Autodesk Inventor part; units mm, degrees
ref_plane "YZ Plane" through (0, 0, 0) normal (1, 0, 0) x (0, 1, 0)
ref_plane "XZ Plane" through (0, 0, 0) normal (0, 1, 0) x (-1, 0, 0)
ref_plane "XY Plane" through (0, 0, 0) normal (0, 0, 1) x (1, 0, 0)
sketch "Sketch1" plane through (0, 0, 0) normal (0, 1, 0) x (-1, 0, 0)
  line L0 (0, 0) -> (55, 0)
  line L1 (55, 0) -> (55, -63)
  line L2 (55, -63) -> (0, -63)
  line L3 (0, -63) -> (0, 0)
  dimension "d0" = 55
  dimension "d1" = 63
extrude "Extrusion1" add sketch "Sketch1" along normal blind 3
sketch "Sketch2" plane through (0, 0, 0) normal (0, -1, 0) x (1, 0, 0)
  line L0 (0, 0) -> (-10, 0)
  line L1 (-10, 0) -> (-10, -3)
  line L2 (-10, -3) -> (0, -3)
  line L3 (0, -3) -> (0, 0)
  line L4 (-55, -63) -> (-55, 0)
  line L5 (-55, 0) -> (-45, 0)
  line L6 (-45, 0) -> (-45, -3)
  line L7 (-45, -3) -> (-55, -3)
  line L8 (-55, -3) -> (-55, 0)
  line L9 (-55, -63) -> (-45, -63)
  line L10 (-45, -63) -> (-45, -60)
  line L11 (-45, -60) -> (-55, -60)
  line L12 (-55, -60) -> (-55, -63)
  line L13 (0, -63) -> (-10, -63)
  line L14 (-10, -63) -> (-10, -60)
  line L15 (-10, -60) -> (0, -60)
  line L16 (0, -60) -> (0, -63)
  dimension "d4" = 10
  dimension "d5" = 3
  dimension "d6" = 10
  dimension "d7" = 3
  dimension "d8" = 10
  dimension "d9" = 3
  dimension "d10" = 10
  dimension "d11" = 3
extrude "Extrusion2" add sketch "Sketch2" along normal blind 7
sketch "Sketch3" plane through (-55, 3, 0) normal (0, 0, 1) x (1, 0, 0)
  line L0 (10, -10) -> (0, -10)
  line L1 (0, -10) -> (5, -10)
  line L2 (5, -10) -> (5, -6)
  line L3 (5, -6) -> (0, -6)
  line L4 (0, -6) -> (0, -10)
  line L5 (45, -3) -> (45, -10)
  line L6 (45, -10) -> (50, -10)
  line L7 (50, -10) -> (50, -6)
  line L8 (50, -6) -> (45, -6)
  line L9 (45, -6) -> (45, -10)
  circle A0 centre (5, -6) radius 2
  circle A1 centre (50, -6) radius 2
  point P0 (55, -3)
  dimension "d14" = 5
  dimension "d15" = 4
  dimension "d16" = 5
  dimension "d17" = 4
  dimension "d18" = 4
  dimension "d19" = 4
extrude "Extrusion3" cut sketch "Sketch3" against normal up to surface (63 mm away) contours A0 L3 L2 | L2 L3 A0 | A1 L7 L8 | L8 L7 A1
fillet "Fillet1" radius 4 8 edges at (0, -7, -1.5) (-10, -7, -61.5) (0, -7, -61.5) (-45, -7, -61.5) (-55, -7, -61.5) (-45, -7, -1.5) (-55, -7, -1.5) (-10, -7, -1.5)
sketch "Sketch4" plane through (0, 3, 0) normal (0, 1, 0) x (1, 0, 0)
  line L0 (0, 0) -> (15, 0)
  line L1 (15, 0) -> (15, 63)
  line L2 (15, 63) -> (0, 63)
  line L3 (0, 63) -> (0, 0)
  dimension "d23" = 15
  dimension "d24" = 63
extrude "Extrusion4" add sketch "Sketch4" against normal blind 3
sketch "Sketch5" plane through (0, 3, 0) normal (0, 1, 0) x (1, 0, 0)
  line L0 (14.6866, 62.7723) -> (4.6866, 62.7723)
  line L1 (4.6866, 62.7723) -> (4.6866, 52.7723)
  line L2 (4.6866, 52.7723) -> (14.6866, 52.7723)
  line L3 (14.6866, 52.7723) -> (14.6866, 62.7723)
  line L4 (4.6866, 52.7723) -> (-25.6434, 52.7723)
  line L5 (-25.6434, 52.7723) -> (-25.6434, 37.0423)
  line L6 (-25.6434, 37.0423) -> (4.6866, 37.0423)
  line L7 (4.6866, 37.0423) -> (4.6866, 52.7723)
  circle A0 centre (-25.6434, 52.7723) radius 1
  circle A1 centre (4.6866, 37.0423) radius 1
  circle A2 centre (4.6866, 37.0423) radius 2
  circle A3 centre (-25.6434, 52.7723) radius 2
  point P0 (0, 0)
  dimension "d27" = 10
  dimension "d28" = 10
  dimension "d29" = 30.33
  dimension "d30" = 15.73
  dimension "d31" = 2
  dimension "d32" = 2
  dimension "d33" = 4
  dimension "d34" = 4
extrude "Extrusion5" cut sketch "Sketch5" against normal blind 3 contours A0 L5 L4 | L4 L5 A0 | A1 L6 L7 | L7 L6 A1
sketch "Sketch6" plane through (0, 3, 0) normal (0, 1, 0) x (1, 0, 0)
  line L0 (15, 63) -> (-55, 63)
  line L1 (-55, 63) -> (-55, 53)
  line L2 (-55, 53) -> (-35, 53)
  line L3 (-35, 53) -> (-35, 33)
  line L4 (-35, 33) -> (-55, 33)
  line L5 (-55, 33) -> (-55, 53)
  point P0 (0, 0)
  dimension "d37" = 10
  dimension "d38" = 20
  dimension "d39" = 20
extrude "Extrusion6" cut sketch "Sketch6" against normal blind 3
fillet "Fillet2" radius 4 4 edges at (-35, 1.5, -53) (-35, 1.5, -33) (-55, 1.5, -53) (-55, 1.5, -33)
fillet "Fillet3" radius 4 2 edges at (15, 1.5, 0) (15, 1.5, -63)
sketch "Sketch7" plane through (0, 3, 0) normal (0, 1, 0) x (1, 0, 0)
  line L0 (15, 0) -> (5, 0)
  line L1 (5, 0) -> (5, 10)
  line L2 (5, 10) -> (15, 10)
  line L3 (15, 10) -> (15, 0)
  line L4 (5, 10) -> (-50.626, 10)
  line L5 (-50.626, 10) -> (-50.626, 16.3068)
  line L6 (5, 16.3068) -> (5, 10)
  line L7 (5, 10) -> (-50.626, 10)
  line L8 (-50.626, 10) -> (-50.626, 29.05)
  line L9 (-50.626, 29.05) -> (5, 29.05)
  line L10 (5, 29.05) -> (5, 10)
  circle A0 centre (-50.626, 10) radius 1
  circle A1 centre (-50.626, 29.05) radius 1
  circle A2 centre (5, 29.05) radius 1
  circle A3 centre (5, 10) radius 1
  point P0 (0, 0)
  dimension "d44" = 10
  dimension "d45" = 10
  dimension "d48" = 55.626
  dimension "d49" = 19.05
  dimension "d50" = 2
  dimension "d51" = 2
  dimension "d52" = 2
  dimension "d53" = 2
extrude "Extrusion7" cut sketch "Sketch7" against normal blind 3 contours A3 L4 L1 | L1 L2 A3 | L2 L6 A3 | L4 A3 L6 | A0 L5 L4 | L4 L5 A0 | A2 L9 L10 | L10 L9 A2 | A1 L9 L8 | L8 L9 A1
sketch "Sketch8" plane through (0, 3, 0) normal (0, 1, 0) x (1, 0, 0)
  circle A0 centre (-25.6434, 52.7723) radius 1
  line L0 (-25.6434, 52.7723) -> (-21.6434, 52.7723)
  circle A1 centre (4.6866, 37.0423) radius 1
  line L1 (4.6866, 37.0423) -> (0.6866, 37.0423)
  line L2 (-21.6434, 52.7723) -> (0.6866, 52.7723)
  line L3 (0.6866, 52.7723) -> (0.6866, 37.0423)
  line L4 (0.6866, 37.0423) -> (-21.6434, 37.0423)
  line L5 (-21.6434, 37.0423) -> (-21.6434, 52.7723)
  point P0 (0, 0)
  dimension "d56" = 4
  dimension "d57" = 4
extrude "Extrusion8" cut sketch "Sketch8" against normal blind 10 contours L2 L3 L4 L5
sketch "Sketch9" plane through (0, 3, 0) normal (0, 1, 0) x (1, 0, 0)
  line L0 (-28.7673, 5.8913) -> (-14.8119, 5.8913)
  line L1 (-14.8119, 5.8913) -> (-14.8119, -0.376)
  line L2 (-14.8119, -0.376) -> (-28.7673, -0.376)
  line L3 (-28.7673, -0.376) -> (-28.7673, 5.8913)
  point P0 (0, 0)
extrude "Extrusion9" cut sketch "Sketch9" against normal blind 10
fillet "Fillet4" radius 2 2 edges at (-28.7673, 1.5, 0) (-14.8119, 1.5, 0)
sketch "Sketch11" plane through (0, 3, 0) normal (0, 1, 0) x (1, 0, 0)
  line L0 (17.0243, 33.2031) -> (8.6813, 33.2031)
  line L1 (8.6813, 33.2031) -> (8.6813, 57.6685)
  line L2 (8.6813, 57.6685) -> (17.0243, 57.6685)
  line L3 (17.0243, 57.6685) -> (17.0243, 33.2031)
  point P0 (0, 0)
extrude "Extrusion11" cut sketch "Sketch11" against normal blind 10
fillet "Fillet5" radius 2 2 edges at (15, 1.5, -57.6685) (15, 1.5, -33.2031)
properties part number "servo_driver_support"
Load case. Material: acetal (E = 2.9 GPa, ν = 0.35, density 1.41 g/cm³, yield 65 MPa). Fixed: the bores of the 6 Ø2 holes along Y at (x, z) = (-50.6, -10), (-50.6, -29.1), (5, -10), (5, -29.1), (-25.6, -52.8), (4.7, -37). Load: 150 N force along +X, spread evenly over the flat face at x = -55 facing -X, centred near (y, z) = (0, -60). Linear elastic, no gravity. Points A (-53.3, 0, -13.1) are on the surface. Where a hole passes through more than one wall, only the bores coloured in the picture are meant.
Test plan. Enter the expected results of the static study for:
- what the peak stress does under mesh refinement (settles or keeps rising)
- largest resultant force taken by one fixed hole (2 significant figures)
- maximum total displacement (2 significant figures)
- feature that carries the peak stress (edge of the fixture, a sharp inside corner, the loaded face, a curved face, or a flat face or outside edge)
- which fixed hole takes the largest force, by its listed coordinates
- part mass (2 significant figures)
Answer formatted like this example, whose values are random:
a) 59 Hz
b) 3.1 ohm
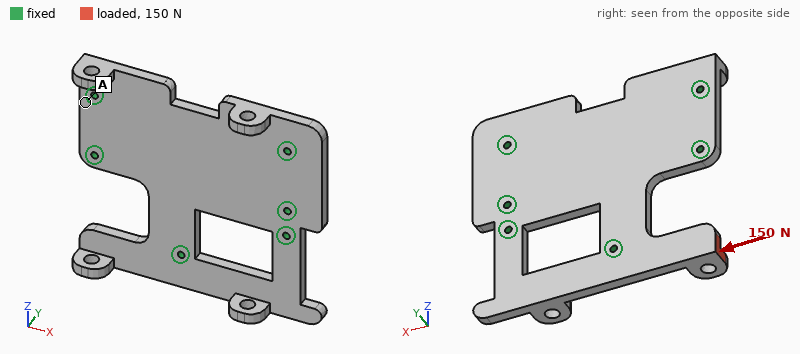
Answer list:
a) keeps rising
b) 160 N
c) 0.93 mm
d) edge of the fixture
e) (-25.6, -52.8)
f) 15 g
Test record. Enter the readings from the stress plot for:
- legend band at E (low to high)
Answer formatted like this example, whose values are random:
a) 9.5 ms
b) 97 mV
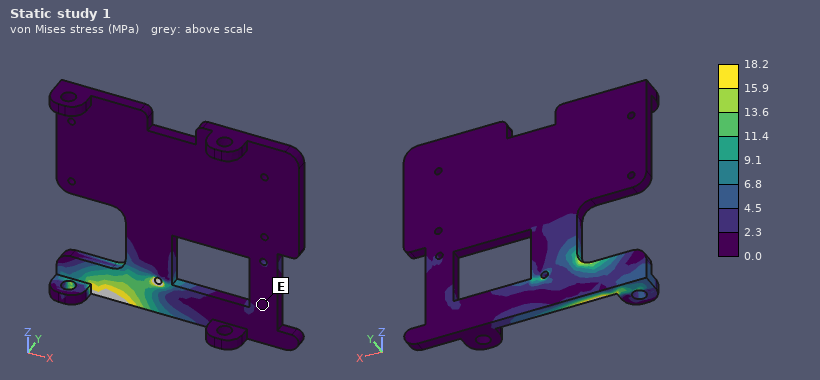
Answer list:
a) 0.0 to 2.3 MPa
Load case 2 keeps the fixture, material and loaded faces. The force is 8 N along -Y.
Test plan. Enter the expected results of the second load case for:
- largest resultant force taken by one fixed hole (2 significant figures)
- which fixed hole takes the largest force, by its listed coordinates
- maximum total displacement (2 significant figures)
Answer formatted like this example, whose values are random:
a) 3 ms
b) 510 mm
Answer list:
a) 10 N
b) (-25.6, -52.8)
c) 0.94 mm
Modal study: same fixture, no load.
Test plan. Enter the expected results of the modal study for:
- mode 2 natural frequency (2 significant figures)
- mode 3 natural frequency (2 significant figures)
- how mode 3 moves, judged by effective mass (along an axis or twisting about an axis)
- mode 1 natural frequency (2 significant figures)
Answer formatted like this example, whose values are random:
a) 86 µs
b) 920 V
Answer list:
a) 960 Hz
b) 1400 Hz
c) along Y
d) 720 Hz
